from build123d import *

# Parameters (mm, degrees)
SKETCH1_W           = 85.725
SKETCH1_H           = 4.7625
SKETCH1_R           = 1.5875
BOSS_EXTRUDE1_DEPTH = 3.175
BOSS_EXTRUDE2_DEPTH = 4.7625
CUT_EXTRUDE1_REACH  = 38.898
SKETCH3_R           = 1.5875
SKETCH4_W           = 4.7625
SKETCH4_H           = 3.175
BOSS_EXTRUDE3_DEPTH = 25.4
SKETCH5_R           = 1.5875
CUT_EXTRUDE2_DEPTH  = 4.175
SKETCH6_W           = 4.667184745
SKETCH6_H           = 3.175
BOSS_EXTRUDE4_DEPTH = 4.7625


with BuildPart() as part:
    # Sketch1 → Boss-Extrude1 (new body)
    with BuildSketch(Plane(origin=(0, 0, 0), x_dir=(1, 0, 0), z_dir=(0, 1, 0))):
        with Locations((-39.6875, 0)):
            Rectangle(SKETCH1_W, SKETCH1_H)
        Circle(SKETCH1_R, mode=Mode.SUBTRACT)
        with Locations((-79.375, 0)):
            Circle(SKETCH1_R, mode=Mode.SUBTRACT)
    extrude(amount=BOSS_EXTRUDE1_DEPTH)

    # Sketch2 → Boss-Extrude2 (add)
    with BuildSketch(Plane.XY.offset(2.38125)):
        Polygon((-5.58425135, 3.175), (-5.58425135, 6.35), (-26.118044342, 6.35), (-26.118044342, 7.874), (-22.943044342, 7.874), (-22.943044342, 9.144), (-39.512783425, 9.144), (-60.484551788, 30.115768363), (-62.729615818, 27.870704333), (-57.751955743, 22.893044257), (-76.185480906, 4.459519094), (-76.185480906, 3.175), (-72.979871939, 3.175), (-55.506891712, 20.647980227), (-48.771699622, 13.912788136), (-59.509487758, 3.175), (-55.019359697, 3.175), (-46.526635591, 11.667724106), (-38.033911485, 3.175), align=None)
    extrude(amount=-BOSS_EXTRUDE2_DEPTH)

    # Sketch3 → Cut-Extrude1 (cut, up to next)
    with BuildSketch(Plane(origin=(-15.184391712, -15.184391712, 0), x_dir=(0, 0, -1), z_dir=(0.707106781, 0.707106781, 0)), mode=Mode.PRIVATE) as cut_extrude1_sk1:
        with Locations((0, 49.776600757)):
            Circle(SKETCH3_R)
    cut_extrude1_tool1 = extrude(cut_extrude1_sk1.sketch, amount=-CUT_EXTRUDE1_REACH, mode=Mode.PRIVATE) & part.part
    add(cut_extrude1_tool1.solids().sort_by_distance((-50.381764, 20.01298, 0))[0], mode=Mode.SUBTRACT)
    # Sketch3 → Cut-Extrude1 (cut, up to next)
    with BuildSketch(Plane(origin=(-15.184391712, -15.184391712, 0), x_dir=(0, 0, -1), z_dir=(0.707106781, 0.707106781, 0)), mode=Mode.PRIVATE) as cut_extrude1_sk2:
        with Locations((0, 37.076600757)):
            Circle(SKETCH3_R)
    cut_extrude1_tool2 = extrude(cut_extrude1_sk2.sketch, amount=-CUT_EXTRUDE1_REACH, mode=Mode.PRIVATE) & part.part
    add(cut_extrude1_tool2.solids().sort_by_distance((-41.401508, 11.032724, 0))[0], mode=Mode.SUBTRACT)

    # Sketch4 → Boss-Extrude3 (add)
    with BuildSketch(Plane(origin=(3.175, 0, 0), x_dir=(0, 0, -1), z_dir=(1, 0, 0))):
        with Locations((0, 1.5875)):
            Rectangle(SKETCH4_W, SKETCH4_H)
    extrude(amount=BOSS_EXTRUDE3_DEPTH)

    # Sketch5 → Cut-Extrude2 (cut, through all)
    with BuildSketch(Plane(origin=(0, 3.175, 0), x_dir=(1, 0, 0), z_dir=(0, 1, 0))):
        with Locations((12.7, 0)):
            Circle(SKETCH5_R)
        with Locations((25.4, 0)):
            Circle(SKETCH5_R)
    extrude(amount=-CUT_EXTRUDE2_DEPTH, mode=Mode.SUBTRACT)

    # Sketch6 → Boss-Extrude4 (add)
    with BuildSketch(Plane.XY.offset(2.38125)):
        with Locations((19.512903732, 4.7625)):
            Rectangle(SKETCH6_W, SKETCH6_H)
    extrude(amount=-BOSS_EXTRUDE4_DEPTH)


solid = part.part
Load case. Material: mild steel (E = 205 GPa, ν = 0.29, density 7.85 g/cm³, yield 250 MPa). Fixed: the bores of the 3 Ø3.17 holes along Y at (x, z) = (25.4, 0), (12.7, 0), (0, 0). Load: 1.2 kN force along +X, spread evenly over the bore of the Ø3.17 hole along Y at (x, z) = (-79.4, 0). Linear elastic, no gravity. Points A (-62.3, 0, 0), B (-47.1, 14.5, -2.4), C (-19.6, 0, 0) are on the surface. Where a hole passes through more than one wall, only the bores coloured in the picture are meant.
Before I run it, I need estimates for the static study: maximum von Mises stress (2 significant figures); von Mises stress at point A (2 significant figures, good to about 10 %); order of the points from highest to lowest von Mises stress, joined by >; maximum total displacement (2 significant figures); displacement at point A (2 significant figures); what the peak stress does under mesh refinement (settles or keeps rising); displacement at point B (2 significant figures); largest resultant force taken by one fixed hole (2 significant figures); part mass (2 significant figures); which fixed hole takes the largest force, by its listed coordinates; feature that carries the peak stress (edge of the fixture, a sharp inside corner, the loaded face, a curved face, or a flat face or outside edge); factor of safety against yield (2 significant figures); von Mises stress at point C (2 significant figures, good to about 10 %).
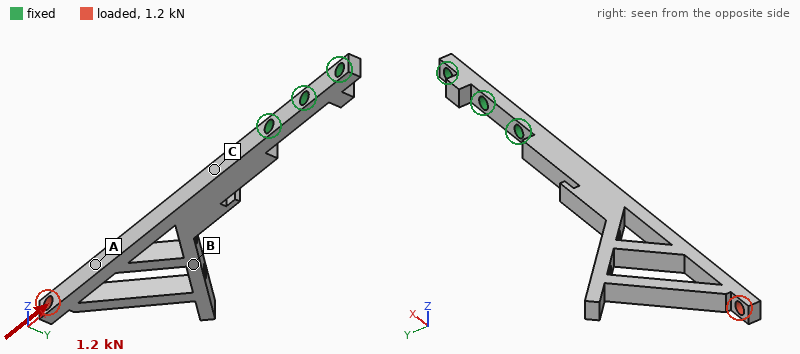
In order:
260 MPa
81 MPa
C > A > B
0.20 mm
0.12 mm
settles
0.073 mm
1.2 kN
27 g
(0, 0)
the loaded face
0.98
99 MPa
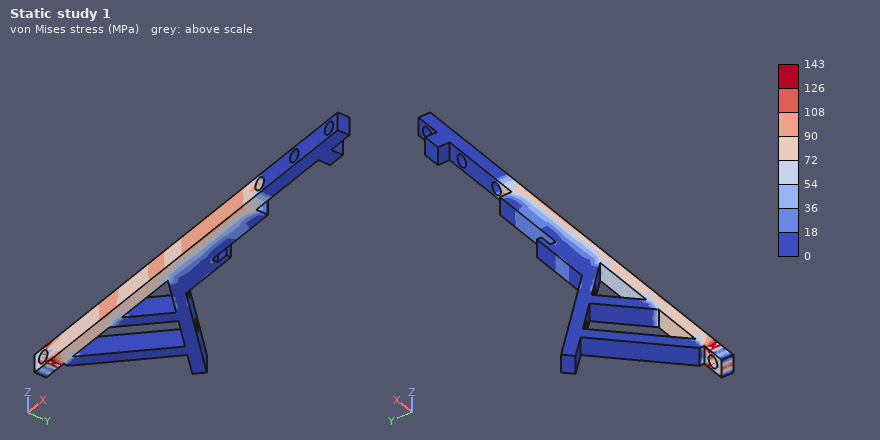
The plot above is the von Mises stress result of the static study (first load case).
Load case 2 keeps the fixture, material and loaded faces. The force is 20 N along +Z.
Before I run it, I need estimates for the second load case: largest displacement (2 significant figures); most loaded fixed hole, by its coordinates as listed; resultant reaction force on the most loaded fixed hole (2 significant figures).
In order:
0.38 mm
(0, 0)
25 N
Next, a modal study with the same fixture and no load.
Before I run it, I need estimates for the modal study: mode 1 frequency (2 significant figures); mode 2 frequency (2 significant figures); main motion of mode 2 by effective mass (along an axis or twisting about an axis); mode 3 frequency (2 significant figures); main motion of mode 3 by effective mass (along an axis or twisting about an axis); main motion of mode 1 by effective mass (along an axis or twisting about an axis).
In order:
440 Hz
480 Hz
along Z
1900 Hz
twisting about X
along Y
